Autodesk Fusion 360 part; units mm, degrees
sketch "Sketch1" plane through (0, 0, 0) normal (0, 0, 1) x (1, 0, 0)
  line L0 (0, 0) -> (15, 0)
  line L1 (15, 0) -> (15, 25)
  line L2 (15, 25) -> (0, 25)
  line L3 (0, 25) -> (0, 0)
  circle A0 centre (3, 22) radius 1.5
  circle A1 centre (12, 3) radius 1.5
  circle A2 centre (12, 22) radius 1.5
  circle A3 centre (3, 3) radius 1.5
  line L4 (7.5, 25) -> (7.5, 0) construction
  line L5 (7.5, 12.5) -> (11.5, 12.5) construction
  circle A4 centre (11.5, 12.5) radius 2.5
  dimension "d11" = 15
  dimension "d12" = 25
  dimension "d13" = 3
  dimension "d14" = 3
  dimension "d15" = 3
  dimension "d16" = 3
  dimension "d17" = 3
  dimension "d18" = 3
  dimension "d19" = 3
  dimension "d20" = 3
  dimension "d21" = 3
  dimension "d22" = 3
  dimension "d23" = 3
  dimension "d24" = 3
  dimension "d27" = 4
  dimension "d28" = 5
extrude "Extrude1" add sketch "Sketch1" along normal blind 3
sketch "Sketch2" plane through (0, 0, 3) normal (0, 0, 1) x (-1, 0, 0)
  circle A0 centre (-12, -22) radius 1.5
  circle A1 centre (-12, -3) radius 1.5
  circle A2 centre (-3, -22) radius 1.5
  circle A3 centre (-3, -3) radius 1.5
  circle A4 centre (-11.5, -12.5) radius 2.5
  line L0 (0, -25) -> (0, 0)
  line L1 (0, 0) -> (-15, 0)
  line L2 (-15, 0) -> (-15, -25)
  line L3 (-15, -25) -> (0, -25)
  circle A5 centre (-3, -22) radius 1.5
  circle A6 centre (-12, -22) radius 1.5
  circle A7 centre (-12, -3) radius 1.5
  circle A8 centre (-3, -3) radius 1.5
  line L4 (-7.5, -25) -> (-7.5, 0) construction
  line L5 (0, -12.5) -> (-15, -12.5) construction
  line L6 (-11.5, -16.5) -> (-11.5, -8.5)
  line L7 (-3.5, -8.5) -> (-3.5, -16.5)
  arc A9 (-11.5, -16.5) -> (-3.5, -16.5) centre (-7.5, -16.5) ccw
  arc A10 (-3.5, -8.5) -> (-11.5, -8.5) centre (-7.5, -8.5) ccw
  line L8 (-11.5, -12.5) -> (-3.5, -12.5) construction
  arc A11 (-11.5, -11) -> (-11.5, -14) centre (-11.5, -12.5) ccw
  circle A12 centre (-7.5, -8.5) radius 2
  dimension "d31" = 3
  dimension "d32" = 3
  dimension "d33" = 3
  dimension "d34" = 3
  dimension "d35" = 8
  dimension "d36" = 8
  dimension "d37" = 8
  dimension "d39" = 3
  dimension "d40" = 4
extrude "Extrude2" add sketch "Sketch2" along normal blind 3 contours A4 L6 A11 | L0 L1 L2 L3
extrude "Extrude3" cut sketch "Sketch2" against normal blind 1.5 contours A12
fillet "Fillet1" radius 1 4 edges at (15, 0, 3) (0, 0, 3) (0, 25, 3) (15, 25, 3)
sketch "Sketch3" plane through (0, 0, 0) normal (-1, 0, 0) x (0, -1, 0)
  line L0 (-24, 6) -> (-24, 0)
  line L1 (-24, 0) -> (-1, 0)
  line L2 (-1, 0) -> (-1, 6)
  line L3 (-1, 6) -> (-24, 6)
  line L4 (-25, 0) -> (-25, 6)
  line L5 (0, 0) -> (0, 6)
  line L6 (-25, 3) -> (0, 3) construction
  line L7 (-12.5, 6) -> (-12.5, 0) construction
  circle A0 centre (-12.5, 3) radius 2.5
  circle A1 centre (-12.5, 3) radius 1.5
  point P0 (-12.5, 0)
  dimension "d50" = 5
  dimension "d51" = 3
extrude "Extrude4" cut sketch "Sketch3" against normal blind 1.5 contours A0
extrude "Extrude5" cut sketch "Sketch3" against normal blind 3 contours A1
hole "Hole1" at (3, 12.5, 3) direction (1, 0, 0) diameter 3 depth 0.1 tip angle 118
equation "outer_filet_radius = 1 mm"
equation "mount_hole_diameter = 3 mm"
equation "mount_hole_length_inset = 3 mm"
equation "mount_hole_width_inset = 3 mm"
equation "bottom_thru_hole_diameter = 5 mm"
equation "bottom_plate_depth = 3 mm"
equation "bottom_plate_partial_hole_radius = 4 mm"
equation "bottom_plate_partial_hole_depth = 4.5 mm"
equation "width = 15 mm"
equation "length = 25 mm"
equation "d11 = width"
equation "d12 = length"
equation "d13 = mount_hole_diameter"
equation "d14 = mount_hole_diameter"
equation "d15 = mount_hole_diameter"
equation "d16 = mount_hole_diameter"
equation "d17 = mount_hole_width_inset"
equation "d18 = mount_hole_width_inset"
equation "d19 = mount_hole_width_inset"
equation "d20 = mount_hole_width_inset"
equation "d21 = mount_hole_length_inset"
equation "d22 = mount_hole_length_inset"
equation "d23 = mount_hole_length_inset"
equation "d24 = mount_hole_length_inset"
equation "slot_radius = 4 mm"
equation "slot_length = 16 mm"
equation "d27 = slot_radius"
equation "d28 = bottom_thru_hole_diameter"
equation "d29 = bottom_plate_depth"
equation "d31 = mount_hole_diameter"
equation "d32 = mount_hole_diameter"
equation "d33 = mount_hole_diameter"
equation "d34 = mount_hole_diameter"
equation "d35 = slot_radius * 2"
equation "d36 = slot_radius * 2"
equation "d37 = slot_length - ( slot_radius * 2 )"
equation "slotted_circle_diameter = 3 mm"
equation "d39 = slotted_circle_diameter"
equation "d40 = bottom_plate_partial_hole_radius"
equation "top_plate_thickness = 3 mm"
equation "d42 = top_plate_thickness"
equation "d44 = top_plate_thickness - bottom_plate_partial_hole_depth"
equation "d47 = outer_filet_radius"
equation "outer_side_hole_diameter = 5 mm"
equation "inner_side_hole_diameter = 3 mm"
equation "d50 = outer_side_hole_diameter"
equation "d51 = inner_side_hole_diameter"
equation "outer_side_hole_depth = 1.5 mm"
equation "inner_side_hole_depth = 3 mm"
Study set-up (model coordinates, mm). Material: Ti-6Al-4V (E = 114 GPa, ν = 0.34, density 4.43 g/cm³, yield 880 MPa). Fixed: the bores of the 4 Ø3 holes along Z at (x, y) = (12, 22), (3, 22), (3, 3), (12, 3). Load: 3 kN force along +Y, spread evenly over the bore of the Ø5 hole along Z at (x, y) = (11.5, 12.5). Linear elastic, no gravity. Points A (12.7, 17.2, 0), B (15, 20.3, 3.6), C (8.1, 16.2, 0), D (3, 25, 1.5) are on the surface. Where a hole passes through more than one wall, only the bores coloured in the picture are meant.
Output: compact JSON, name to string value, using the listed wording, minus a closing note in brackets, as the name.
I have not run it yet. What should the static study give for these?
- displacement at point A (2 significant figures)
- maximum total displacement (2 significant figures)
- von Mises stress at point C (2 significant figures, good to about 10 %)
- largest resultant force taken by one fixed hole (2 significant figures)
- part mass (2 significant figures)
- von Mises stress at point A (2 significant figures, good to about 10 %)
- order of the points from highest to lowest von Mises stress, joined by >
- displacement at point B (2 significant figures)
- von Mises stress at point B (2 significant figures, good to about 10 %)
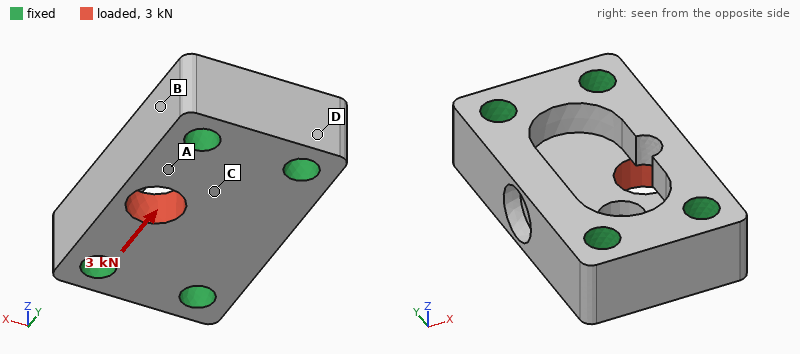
{"displacement at point A": "2.0 µm", "maximum total displacement": "4.4 µm", "von Mises stress at point C": "40 MPa", "largest resultant force taken by one fixed hole": "1.2 kN", "part mass": "7.1 g", "von Mises stress at point A": "67 MPa", "order of the points from highest to lowest von Mises stress, joined by >": "A > C > B > D", "displacement at point B": "0.72 µm", "von Mises stress at point B": "25 MPa"}
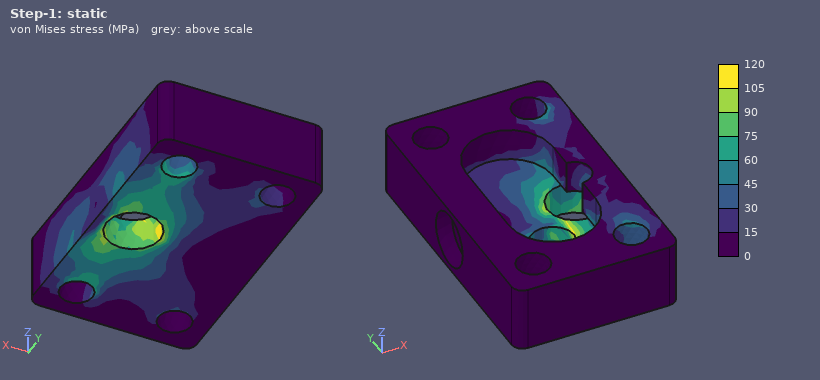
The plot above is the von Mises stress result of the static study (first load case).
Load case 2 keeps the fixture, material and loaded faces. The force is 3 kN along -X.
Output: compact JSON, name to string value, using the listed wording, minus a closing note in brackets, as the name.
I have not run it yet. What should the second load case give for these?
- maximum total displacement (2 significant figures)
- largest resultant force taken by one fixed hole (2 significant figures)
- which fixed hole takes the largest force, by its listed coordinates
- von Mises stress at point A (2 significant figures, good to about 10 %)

{"maximum total displacement": "18 µm", "largest resultant force taken by one fixed hole": "1.0 kN", "which fixed hole takes the largest force, by its listed coordinates": "(3, 22)", "von Mises stress at point A": "78 MPa"}
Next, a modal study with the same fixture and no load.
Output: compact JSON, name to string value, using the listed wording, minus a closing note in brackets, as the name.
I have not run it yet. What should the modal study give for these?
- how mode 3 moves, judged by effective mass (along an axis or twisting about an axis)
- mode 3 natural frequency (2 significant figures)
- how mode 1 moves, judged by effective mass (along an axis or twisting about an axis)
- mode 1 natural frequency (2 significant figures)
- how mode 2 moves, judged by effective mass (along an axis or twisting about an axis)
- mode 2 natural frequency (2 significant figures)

{"how mode 3 moves, judged by effective mass": "along X", "mode 3 natural frequency": "80 kHz", "how mode 1 moves, judged by effective mass": "along Z", "mode 1 natural frequency": "65 kHz", "how mode 2 moves, judged by effective mass": "along X", "mode 2 natural frequency": "73 kHz"}
